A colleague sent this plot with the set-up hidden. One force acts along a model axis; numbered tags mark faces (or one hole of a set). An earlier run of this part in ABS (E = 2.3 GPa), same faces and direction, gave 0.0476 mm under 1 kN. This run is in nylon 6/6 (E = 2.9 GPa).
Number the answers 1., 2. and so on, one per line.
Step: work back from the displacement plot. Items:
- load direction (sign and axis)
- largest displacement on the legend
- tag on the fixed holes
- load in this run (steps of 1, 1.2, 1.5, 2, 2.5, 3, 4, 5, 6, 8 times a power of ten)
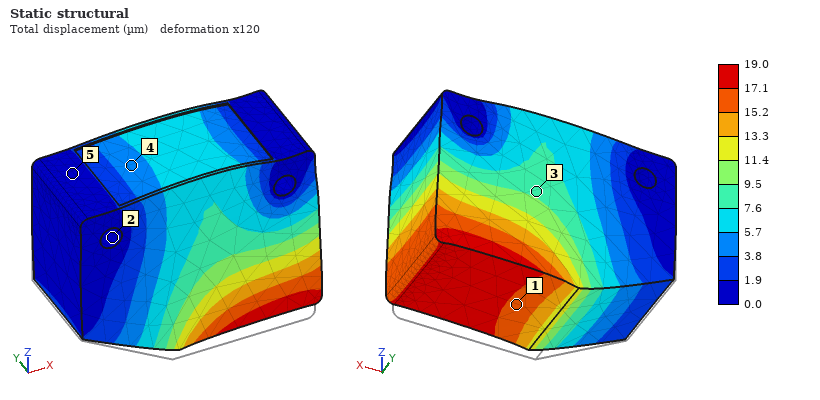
1. +Z
2. 19.0 µm
3. 2
4. 500 N
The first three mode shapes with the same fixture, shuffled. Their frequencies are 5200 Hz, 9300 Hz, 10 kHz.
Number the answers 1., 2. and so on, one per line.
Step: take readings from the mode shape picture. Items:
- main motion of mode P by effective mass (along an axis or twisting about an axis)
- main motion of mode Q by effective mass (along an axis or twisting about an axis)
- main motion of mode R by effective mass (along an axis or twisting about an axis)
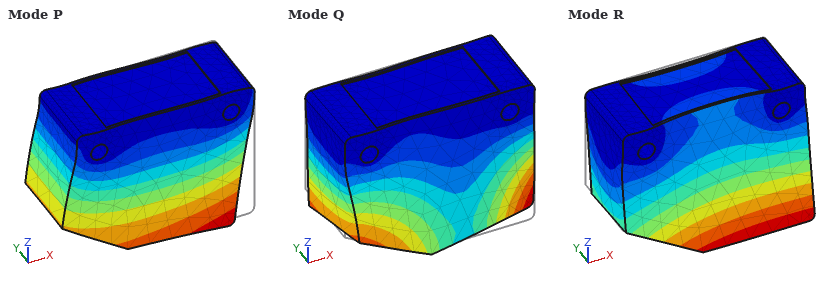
1. along X
2. twisting about Z
3. along Y
